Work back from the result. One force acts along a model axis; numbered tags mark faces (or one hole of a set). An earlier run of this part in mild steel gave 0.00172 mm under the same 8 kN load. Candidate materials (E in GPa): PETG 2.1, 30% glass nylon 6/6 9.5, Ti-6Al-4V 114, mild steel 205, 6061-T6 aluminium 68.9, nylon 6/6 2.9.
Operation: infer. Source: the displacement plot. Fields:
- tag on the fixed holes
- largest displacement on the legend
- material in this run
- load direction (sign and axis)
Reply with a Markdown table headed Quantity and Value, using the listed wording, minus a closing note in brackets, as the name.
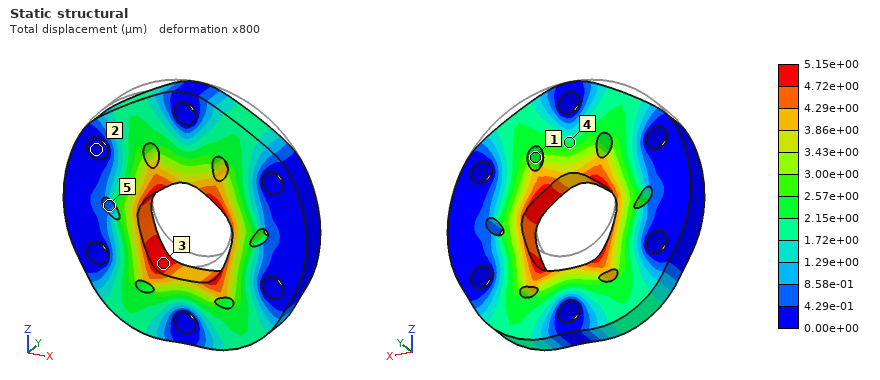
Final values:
| Quantity | Value |
|---|---|
| tag on the fixed holes | 2 |
| largest displacement on the legend | 5.15e+00 µm |
| material in this run | 6061-T6 aluminium |
| load direction | -Z |
